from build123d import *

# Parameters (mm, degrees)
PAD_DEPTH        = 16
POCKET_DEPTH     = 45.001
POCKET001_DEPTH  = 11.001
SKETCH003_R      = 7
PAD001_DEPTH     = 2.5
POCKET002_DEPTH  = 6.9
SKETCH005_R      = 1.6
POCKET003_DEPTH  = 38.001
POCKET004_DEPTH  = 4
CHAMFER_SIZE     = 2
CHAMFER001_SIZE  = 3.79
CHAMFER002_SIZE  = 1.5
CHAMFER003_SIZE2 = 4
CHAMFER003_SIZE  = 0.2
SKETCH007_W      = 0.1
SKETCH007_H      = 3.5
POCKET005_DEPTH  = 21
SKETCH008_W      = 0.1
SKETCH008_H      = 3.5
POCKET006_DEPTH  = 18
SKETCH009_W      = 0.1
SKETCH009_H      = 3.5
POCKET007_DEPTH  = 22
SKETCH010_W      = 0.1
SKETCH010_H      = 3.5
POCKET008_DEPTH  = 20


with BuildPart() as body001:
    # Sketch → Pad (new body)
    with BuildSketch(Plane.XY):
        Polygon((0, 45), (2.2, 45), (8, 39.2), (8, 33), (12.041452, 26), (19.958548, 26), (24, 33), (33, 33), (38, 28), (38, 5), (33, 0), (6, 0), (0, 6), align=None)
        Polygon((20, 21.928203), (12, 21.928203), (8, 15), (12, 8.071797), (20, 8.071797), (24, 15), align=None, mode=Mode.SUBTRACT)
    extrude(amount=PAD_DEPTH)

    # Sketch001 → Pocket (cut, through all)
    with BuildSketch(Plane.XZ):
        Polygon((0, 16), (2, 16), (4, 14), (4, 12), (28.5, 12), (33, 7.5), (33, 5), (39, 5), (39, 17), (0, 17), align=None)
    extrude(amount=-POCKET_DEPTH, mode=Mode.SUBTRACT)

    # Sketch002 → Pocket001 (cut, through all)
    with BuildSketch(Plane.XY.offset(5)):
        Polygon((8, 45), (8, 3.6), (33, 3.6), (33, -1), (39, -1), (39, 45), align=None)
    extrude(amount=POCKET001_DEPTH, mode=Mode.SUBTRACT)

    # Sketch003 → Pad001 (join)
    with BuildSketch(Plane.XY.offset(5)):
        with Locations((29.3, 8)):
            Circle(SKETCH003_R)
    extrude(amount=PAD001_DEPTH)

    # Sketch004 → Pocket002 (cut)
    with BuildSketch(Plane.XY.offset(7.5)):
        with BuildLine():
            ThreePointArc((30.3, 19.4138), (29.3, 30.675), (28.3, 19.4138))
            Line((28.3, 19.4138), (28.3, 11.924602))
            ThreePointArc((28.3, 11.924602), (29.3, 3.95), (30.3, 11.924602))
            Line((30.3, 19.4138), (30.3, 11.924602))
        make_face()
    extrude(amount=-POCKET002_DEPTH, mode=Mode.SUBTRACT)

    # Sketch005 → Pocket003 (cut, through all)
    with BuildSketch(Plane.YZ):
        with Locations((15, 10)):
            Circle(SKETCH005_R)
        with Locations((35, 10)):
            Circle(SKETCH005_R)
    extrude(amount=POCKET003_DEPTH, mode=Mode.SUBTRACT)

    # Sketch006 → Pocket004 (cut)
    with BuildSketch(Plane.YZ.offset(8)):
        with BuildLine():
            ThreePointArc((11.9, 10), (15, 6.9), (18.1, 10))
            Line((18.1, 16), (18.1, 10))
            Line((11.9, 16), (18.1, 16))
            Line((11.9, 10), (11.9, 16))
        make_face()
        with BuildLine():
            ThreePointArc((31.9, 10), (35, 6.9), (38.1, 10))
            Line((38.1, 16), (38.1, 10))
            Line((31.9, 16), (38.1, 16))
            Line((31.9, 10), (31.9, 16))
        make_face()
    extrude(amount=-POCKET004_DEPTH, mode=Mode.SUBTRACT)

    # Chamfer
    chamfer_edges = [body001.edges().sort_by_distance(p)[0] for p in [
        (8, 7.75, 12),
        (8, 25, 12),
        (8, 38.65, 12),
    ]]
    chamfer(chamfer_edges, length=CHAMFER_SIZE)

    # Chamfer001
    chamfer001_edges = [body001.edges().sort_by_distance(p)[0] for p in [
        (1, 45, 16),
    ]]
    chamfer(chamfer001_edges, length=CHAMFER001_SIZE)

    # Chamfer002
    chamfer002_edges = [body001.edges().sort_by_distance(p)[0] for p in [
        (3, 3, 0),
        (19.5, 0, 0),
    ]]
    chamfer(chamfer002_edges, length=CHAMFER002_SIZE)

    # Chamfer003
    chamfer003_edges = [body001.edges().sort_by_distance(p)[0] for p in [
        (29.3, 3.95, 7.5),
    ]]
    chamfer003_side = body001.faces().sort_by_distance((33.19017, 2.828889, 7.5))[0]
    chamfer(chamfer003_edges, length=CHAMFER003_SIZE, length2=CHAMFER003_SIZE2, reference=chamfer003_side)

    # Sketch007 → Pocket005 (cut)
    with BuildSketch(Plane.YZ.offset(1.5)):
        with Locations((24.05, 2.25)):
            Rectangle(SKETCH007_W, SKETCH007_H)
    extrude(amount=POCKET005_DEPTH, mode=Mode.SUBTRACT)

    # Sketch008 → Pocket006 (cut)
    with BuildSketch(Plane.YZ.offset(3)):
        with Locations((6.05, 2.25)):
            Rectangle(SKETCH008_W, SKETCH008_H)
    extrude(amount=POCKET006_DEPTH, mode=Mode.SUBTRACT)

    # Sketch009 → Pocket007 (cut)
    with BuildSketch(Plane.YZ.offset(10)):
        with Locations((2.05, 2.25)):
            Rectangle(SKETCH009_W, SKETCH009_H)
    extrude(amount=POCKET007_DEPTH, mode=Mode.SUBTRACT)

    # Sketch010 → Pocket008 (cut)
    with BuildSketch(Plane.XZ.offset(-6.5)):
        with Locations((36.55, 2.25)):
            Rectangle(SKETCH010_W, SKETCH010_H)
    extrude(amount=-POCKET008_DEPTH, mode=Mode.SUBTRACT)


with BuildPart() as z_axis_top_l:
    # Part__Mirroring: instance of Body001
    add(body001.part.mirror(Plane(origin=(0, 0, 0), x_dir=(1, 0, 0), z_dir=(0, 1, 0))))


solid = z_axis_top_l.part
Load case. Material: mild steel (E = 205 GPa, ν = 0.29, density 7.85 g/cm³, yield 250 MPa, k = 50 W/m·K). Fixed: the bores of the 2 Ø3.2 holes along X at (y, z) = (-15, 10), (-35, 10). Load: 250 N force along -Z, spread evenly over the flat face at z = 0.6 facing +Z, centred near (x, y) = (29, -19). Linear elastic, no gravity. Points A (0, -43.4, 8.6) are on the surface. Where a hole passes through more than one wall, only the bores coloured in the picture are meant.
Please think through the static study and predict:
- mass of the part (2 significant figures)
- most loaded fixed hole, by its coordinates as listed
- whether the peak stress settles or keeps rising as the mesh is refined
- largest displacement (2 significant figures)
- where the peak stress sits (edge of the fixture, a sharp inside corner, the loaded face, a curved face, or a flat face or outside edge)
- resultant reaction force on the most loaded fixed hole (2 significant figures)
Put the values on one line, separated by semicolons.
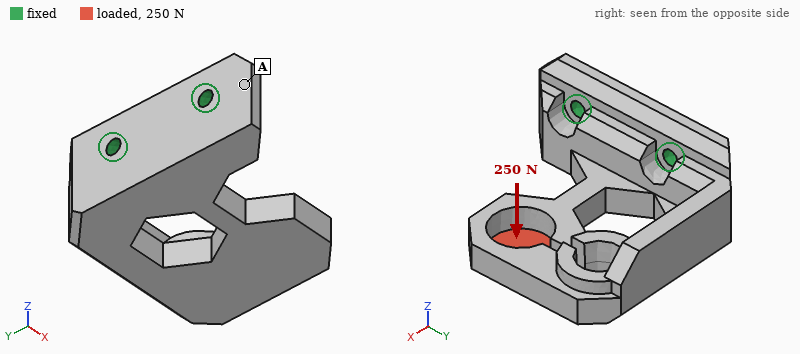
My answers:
60 g; (-15, 10); keeps rising; 67 µm; edge of the fixture; 190 N
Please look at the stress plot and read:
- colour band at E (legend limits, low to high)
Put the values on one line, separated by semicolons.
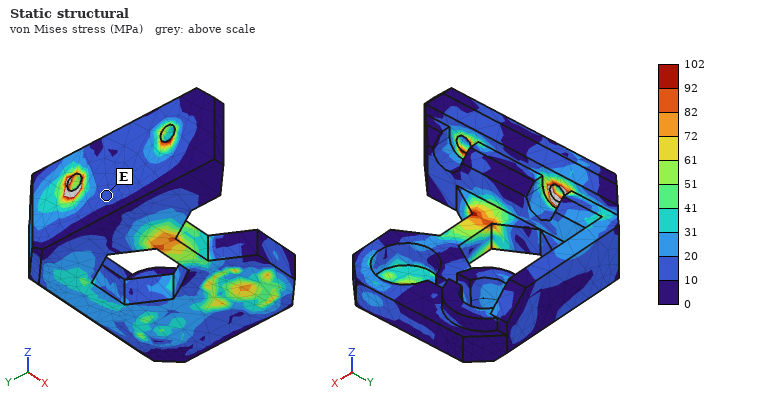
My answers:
10 to 20 MPa
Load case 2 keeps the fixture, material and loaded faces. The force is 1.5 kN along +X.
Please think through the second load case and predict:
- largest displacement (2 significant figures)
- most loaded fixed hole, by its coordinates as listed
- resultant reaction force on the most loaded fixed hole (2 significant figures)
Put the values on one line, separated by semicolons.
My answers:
75 µm; (-15, 10); 1.2 kN
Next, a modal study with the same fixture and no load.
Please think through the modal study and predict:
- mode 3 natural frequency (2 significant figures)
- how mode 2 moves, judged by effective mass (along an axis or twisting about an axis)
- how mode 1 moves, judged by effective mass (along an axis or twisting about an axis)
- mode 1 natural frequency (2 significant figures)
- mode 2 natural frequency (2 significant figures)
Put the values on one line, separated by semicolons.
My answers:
7100 Hz; along Y; along Z; 2800 Hz; 4700 Hz
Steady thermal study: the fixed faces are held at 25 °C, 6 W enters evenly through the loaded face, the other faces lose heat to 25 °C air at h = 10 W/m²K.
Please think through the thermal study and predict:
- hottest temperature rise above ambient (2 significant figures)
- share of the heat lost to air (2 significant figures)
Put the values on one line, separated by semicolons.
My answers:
51 K; 16 %
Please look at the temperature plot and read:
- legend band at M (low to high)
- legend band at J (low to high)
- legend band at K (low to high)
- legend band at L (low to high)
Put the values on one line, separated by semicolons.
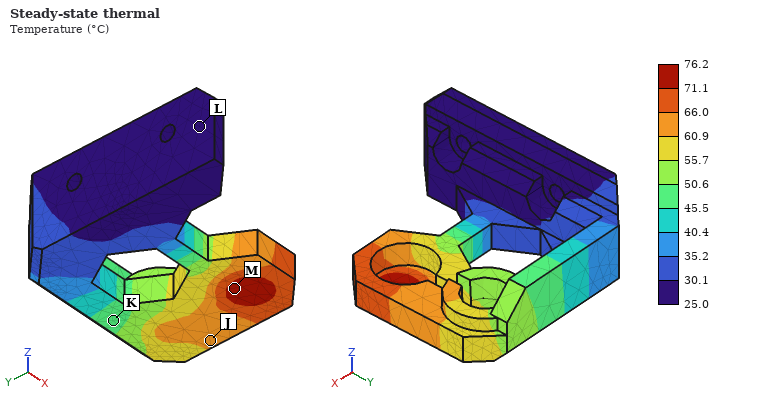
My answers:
71.1 to 76.2 °C; 60.9 to 66.0 °C; 45.5 to 50.6 °C; 25.0 to 30.1 °C
